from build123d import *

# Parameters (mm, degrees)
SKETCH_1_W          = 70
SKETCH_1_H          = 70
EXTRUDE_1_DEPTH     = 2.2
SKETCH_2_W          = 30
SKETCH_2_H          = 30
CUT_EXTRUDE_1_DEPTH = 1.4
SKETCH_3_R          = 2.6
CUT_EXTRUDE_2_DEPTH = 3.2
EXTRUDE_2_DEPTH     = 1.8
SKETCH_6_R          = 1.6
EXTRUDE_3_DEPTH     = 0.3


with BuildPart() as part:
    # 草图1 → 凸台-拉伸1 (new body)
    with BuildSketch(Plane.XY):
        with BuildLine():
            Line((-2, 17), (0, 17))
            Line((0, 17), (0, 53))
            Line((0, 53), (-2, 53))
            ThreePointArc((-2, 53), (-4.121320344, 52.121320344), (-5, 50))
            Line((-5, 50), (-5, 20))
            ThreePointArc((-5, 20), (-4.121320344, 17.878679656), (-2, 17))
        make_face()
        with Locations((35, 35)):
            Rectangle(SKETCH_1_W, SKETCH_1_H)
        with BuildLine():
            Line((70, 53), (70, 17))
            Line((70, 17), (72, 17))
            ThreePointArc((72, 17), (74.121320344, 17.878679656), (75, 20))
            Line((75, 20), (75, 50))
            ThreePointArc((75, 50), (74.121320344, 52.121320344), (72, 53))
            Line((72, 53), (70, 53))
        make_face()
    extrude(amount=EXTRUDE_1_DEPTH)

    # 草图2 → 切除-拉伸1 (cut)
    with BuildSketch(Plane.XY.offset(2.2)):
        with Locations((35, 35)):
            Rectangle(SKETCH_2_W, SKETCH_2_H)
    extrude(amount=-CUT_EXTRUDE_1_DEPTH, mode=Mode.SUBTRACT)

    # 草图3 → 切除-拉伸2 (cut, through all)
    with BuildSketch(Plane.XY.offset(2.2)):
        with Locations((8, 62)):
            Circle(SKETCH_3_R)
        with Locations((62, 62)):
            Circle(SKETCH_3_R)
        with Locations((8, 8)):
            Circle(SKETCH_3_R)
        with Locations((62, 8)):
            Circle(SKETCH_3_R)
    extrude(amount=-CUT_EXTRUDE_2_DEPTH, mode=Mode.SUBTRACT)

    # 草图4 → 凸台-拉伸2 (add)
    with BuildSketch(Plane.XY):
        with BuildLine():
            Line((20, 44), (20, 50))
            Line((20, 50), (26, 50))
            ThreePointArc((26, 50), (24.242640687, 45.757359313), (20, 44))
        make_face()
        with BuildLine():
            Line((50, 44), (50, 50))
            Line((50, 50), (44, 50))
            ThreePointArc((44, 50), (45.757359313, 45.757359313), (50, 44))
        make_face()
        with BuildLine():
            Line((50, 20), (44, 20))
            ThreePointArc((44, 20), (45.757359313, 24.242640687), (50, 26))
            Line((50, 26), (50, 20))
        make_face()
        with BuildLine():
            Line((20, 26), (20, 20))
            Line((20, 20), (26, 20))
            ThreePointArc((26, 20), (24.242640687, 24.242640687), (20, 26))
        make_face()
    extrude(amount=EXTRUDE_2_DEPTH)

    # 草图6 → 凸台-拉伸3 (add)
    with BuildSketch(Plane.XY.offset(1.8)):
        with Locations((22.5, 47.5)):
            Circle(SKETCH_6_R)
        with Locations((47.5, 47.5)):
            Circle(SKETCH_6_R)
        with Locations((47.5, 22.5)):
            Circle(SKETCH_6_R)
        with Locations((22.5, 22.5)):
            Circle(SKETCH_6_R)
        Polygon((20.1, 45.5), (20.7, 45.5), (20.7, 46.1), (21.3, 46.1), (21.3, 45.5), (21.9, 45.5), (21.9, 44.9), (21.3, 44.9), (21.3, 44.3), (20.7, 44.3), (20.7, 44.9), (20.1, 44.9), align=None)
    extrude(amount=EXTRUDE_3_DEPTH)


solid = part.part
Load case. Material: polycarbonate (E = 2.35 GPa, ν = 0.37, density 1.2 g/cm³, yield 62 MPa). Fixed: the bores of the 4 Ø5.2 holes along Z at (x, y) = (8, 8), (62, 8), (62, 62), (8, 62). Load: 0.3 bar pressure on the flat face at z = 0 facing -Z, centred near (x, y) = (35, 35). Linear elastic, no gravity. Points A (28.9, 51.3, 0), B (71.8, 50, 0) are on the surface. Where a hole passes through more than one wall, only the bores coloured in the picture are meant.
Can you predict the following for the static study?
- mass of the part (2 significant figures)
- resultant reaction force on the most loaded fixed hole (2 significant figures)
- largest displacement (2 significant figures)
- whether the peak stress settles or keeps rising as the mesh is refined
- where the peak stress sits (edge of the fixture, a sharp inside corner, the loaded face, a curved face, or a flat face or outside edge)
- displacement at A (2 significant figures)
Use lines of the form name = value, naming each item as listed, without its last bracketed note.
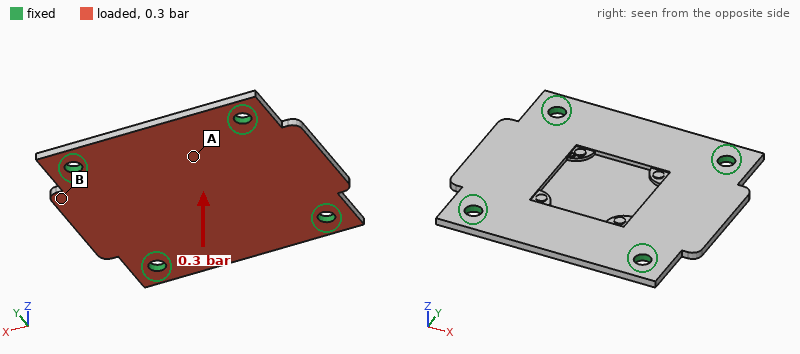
mass of the part = 12 g
resultant reaction force on the most loaded fixed hole = 47 N
largest displacement = 1.1 mm
whether the peak stress settles or keeps rising as the mesh is refined = keeps rising
where the peak stress sits = edge of the fixture
displacement at A = 0.56 mm
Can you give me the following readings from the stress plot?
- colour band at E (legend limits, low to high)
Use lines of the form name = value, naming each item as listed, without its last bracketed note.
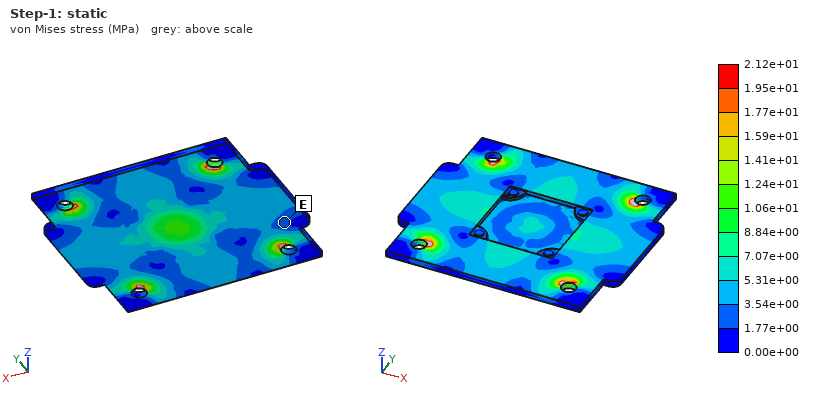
colour band at E = 1.77e+00 to 3.54e+00 MPa
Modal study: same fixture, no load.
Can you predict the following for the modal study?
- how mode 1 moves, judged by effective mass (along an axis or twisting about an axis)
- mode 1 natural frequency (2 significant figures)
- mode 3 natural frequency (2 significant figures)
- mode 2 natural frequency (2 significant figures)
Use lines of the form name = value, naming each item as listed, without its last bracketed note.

how mode 1 moves, judged by effective mass = along Z
mode 1 natural frequency = 910 Hz
mode 3 natural frequency = 1100 Hz
mode 2 natural frequency = 1100 Hz
